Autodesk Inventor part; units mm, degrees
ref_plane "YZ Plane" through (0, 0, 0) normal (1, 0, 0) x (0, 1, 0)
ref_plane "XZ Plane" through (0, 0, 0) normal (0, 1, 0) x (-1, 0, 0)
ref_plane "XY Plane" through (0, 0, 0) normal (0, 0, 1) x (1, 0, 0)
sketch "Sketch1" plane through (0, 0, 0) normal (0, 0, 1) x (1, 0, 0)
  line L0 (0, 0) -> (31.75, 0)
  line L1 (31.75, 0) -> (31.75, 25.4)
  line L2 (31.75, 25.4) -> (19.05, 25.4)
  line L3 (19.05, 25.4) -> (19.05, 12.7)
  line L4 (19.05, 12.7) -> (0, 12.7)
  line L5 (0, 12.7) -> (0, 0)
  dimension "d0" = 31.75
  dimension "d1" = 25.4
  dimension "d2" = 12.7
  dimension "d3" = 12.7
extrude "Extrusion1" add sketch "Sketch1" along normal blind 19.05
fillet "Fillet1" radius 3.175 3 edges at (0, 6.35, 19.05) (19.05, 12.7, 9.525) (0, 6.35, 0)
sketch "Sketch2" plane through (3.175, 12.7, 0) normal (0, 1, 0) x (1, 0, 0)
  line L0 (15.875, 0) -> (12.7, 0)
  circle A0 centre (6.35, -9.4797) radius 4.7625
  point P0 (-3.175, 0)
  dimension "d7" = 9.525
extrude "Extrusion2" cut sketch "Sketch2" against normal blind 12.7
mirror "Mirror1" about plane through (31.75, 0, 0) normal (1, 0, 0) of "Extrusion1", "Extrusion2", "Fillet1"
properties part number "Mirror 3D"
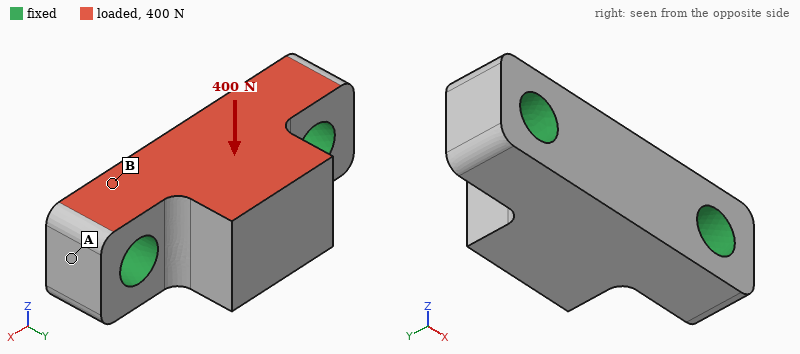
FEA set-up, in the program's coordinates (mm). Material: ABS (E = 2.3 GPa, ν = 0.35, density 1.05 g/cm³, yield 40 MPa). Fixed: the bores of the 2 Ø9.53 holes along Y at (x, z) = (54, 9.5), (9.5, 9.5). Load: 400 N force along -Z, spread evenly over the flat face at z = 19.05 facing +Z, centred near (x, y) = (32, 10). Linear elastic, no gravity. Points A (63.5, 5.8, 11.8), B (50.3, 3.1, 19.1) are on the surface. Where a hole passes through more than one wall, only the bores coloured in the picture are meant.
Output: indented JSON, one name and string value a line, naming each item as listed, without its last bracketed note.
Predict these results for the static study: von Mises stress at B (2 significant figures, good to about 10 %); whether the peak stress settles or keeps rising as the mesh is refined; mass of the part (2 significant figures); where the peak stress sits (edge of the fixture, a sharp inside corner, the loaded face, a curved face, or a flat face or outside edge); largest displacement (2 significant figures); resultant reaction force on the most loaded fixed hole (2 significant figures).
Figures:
{
  "von Mises stress at B": "1.1 MPa",
  "whether the peak stress settles or keeps rising as the mesh is refined": "keeps rising",
  "mass of the part": "21 g",
  "where the peak stress sits": "edge of the fixture",
  "largest displacement": "38 µm",
  "resultant reaction force on the most loaded fixed hole": "200 N"
}
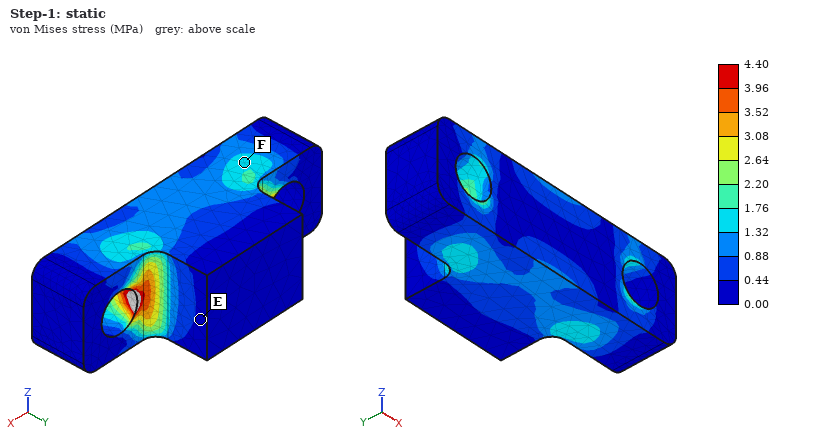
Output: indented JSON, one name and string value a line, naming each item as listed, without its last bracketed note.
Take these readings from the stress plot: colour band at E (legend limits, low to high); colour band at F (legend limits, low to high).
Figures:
{
  "colour band at E": "0.00 to 0.44 MPa",
  "colour band at F": "1.32 to 1.76 MPa"
}
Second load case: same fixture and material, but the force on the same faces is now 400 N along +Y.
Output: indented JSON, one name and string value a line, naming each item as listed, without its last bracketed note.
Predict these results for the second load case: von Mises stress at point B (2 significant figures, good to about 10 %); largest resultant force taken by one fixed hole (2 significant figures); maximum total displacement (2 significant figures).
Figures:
{
  "von Mises stress at point B": "2.1 MPa",
  "largest resultant force taken by one fixed hole": "200 N",
  "maximum total displacement": "50 µm"
}
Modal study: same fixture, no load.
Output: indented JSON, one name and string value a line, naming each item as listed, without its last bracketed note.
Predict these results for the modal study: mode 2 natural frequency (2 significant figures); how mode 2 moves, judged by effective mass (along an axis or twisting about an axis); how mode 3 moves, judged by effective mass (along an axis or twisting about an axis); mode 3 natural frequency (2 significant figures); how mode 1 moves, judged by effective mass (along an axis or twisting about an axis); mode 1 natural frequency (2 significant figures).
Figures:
{
  "mode 2 natural frequency": "7300 Hz",
  "how mode 2 moves, judged by effective mass": "along Y",
  "how mode 3 moves, judged by effective mass": "along Z",
  "mode 3 natural frequency": "8800 Hz",
  "how mode 1 moves, judged by effective mass": "along Z",
  "mode 1 natural frequency": "4300 Hz"
}
